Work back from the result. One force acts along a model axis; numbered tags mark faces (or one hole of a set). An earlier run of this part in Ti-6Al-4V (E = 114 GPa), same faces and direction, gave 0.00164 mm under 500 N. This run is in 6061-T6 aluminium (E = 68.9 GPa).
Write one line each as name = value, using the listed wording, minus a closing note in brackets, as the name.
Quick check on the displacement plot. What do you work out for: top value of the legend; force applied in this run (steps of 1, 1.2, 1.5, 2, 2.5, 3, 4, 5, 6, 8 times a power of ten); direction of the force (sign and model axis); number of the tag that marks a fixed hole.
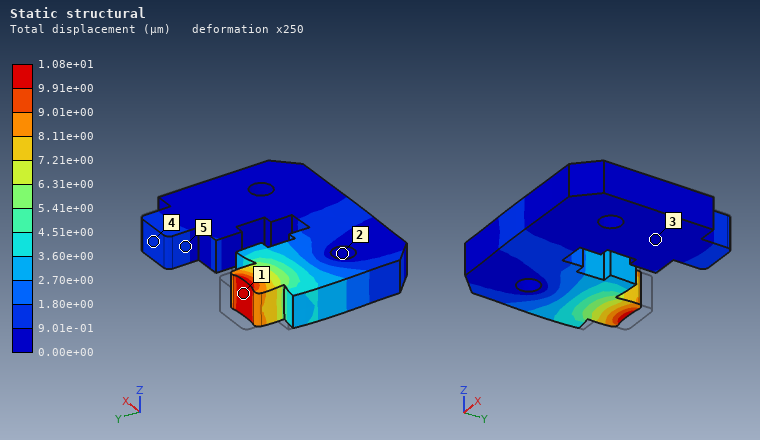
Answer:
top value of the legend = 1.08e+01 µm
force applied in this run = 2 kN
direction of the force = -Y
number of the tag that marks a fixed hole = 2
